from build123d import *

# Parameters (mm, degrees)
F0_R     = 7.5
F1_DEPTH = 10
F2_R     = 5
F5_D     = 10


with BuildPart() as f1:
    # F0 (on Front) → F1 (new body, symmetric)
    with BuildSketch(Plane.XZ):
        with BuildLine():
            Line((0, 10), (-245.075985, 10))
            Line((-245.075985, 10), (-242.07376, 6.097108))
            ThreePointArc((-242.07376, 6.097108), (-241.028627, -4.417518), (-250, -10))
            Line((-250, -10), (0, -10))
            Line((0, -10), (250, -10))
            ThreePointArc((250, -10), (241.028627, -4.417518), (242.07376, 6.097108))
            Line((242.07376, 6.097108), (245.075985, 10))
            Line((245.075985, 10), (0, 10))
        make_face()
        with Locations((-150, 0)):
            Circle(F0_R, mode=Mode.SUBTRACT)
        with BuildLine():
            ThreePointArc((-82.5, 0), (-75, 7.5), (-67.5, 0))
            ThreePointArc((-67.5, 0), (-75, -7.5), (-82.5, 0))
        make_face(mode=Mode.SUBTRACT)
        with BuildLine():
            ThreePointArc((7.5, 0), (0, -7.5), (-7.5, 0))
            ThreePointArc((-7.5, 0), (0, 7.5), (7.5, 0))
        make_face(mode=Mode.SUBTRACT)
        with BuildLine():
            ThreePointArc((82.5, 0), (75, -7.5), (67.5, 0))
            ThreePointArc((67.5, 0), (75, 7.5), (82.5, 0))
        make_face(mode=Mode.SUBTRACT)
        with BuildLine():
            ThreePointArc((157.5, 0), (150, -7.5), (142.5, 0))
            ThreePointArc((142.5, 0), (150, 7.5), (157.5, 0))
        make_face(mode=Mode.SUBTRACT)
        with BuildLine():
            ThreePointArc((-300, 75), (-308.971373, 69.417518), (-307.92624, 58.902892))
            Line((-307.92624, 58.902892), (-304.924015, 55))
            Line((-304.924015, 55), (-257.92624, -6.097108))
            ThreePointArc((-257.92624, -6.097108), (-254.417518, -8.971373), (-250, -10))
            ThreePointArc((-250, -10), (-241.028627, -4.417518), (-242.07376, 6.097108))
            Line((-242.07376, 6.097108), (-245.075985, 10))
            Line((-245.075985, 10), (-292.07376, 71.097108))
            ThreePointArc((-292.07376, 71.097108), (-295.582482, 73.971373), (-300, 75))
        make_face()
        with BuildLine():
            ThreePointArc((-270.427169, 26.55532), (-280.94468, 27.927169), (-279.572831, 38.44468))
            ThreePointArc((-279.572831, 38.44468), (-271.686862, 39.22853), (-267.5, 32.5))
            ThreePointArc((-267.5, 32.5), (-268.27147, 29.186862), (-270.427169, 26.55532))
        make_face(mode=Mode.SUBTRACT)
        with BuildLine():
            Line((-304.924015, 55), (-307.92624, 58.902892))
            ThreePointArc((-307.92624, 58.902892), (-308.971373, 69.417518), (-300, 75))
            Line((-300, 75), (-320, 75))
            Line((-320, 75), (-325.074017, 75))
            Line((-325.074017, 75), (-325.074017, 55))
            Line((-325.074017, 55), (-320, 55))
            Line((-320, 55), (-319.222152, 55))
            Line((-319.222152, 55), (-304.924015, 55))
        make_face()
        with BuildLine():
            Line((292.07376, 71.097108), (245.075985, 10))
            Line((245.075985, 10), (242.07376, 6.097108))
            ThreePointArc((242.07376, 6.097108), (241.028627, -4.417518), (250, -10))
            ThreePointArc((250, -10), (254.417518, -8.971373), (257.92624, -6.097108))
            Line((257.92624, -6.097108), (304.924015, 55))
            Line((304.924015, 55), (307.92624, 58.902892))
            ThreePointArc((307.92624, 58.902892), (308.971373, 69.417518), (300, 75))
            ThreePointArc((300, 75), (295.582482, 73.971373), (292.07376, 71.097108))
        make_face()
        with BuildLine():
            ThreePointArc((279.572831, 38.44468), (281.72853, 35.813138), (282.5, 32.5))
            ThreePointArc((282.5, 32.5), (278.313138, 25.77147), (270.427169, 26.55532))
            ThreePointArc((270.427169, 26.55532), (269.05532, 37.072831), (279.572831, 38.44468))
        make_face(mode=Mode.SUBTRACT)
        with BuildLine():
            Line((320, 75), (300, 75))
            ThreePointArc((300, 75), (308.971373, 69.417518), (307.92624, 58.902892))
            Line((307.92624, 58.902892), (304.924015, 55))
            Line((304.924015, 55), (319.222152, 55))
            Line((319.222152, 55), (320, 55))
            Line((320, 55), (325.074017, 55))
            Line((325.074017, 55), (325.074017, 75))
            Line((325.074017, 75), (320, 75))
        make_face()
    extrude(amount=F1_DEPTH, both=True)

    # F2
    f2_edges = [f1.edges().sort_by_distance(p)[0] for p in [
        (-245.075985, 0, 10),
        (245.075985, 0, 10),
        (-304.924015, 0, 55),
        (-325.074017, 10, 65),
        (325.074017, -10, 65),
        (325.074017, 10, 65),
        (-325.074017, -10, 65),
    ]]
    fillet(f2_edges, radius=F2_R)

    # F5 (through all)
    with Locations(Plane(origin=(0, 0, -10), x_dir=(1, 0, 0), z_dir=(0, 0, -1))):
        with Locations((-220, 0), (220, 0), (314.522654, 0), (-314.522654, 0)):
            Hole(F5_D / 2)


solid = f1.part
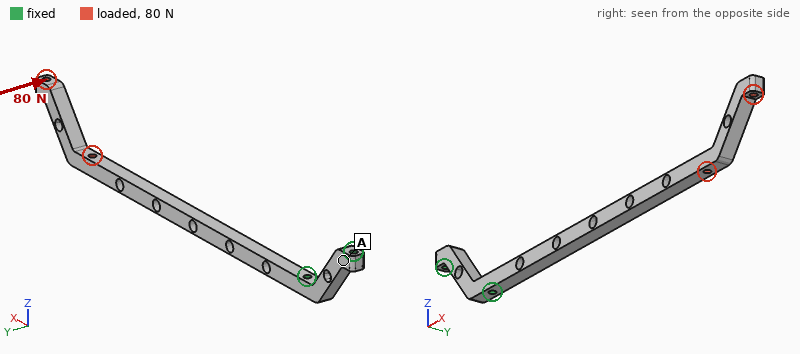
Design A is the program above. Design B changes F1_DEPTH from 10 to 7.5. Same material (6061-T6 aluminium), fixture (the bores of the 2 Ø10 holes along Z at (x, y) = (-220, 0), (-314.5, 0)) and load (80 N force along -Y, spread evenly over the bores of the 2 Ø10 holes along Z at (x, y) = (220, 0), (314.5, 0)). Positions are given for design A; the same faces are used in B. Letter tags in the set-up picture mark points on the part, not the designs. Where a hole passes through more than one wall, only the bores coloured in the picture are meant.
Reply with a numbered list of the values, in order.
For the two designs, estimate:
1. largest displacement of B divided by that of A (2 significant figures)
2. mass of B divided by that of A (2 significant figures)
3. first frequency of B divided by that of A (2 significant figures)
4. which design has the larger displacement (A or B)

1. 2.3
2. 0.74
3. 0.77
4. B
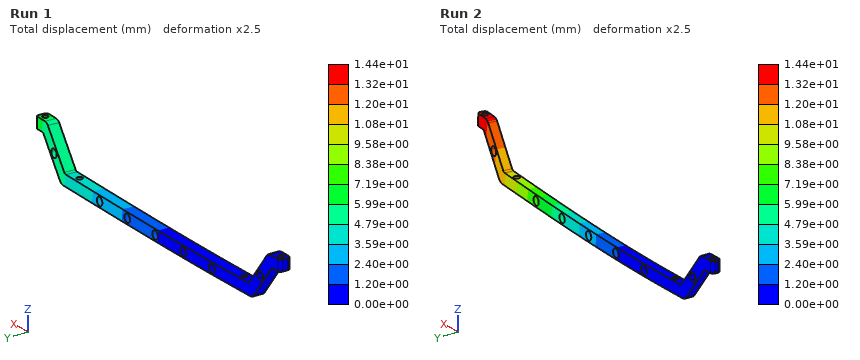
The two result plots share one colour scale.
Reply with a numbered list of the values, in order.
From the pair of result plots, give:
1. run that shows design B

1. Run 2
